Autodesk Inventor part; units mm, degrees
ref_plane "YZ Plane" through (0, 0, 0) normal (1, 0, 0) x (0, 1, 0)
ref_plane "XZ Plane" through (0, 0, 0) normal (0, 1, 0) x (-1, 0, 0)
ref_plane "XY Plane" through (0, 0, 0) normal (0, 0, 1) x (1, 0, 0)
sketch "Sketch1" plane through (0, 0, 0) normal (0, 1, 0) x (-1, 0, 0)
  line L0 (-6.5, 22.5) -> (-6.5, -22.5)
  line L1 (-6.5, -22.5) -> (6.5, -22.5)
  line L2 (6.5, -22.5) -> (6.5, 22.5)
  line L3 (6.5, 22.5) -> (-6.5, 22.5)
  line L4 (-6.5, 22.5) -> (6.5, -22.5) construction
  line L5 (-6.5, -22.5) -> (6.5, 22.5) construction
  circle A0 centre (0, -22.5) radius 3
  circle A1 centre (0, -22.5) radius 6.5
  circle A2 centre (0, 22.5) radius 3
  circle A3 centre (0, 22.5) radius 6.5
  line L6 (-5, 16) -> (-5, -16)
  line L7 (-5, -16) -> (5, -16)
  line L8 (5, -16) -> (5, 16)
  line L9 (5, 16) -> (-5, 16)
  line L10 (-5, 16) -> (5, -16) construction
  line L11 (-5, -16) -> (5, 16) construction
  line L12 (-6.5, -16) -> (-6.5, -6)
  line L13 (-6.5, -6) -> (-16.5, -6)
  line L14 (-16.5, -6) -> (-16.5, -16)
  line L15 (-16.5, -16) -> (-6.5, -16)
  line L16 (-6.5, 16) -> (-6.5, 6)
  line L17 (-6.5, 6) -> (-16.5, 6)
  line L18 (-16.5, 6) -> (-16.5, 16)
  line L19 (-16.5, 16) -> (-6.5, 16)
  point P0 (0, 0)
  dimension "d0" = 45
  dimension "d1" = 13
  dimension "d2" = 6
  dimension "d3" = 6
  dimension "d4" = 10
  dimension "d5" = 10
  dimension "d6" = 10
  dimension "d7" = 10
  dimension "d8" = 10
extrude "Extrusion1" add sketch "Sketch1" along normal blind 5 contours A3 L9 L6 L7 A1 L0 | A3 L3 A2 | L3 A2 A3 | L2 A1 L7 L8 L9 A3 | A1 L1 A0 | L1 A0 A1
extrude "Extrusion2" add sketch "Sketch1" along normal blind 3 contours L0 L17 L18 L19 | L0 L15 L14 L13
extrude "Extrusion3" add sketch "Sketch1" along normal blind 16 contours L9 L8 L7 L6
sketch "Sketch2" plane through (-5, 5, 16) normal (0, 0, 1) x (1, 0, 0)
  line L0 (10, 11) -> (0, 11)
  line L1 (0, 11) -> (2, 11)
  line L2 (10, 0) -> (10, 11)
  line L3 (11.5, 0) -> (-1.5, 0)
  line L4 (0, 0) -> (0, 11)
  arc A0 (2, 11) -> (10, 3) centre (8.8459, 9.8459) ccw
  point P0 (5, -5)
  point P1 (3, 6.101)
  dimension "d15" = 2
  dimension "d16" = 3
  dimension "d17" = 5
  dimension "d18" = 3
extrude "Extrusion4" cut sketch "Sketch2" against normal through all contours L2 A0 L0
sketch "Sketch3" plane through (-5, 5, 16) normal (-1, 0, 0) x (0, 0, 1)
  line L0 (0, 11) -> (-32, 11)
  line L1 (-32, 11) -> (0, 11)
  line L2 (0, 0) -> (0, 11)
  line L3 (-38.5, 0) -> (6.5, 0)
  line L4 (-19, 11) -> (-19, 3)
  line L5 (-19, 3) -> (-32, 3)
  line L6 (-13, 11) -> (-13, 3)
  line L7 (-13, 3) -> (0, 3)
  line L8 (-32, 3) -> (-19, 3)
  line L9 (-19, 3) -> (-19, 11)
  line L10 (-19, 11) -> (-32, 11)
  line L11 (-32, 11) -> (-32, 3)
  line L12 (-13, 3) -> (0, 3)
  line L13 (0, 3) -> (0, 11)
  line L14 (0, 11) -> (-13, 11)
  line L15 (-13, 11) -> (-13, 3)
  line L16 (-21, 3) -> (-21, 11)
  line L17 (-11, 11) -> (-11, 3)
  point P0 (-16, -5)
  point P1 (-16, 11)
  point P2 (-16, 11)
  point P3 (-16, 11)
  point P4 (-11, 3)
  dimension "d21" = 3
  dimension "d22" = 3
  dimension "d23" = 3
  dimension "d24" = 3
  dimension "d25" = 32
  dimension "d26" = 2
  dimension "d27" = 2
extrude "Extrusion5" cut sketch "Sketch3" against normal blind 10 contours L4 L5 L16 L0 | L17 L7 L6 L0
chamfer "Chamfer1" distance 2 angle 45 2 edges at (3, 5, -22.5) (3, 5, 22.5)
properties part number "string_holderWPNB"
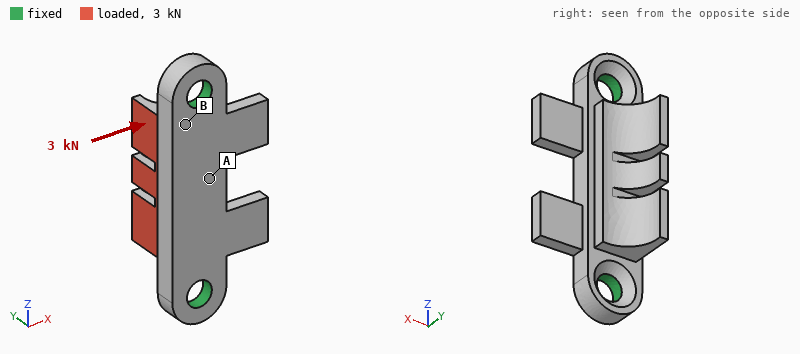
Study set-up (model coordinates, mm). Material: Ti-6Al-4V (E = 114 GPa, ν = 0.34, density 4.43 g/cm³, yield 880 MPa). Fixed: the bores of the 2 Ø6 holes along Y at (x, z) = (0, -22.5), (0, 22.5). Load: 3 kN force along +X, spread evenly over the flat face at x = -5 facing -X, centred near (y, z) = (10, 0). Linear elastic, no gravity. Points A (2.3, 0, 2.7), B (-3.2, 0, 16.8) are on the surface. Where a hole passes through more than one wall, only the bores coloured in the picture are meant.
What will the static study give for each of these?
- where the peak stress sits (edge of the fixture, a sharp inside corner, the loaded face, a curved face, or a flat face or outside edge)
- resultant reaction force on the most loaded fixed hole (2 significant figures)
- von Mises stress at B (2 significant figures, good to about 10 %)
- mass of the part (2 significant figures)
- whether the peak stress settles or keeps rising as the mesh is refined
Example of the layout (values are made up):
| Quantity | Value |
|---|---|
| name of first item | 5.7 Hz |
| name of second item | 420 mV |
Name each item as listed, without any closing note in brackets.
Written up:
| Quantity | Value |
|---|---|
| where the peak stress sits | edge of the fixture |
| resultant reaction force on the most loaded fixed hole | 1.5 kN |
| von Mises stress at B | 97 MPa |
| mass of the part | 24 g |
| whether the peak stress settles or keeps rising as the mesh is refined | keeps rising |
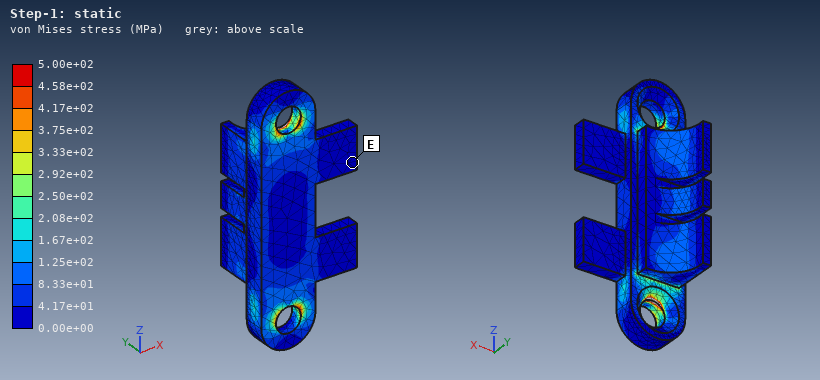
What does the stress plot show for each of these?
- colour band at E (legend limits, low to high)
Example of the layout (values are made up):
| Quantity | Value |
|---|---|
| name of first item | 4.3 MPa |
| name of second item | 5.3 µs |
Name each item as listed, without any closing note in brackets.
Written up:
| Quantity | Value |
|---|---|
| colour band at E | 0.00e+00 to 4.17e+01 MPa |
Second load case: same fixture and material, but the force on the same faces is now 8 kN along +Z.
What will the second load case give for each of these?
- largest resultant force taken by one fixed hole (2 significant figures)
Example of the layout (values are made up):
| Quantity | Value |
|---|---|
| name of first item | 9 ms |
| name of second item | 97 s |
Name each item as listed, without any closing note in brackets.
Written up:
| Quantity | Value |
|---|---|
| largest resultant force taken by one fixed hole | 4.5 kN |
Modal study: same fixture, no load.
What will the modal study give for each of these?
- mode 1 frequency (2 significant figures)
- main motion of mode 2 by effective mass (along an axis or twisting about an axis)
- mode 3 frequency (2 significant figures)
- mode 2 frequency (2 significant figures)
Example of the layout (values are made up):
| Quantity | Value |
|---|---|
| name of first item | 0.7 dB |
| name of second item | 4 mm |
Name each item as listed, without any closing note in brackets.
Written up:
| Quantity | Value |
|---|---|
| mode 1 frequency | 9900 Hz |
| main motion of mode 2 by effective mass | along Y |
| mode 3 frequency | 15 kHz |
| mode 2 frequency | 13 kHz |
